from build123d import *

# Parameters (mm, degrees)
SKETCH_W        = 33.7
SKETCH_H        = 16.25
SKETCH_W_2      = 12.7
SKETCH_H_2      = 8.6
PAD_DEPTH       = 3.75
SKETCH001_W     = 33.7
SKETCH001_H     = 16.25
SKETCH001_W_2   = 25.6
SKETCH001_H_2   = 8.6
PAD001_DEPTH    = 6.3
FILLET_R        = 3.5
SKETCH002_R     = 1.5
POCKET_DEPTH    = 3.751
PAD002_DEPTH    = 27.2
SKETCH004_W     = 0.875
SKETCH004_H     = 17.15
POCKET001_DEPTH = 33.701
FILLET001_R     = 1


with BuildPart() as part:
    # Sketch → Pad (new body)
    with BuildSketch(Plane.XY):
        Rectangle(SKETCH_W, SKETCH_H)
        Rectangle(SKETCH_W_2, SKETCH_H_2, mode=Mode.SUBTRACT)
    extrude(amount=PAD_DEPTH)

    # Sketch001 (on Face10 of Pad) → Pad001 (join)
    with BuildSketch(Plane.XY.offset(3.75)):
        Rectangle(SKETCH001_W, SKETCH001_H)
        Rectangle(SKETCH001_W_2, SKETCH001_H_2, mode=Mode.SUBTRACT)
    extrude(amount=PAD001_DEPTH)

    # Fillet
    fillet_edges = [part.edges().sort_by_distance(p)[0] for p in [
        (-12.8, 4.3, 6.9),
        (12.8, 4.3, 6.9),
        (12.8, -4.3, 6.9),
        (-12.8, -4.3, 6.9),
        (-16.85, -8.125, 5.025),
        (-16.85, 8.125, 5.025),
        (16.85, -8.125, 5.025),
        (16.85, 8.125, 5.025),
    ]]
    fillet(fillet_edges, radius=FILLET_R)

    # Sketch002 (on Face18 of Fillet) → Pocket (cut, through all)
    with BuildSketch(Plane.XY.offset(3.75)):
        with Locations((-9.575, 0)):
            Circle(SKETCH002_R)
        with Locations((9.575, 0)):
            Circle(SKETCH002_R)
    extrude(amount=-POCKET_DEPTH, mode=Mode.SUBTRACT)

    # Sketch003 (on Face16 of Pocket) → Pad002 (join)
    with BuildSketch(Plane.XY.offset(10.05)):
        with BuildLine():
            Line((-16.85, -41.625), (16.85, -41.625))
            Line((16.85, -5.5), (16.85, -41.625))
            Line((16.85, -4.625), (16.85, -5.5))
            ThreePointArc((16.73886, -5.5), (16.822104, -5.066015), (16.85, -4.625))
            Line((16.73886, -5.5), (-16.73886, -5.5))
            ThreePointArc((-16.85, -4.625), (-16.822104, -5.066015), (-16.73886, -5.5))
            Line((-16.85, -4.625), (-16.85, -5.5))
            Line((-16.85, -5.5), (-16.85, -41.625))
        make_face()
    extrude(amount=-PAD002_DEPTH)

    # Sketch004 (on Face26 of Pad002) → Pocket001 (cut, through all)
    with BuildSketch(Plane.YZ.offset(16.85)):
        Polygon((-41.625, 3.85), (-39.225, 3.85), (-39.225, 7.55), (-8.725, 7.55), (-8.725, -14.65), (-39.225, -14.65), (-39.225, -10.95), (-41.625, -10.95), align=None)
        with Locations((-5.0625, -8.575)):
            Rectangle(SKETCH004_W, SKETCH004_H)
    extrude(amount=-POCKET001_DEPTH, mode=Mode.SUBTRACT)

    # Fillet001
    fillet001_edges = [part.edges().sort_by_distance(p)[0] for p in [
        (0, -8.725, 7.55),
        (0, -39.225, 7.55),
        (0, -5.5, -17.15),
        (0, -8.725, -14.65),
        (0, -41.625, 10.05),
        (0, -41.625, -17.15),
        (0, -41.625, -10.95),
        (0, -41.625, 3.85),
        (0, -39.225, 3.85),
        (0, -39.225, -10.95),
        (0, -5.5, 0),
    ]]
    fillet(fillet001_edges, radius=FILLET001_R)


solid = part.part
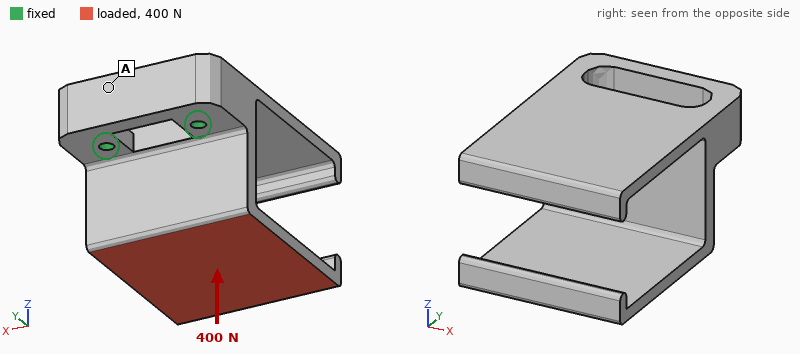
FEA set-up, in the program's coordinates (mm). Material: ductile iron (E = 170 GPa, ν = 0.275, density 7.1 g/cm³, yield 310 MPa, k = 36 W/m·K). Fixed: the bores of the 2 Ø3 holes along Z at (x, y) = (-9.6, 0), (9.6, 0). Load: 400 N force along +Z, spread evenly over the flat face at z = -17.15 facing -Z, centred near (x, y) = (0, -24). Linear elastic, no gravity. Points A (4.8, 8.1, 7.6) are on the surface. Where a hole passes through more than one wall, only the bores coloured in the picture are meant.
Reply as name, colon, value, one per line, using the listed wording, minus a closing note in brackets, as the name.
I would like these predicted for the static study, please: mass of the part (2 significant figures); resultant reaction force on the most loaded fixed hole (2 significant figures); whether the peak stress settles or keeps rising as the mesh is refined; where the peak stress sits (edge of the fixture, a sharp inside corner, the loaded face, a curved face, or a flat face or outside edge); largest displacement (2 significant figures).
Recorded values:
mass of the part: 84 g
resultant reaction force on the most loaded fixed hole: 210 N
whether the peak stress settles or keeps rising as the mesh is refined: keeps rising
where the peak stress sits: edge of the fixture
largest displacement: 0.50 mm
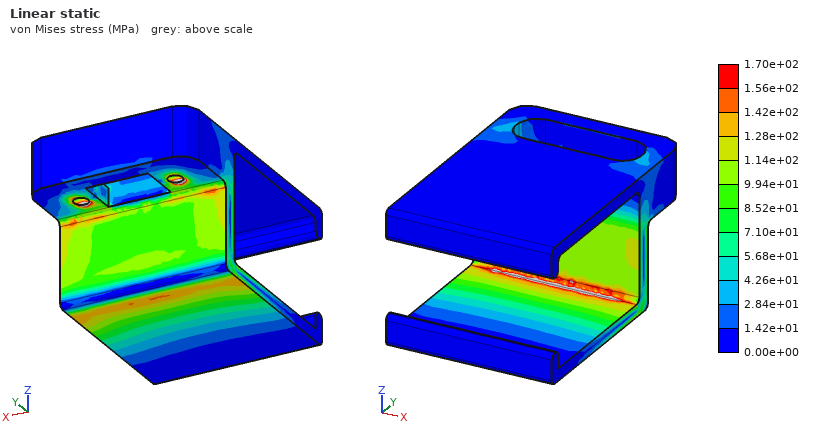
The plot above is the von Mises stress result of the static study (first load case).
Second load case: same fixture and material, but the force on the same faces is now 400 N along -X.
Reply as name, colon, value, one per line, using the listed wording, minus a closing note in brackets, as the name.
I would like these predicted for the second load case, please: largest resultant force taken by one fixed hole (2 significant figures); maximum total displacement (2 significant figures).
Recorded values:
largest resultant force taken by one fixed hole: 570 N
maximum total displacement: 88 µm
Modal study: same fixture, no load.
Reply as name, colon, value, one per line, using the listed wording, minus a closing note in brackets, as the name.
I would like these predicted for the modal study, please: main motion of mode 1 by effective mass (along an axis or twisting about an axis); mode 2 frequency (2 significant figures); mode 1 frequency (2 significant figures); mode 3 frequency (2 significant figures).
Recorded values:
main motion of mode 1 by effective mass: along Z
mode 2 frequency: 1400 Hz
mode 1 frequency: 1000 Hz
mode 3 frequency: 2300 Hz
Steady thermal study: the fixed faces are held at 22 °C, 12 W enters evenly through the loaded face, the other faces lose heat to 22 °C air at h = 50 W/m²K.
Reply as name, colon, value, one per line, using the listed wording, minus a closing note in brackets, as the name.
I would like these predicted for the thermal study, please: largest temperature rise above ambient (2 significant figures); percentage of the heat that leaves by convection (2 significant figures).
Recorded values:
largest temperature rise above ambient: 65 K
percentage of the heat that leaves by convection: 60 %
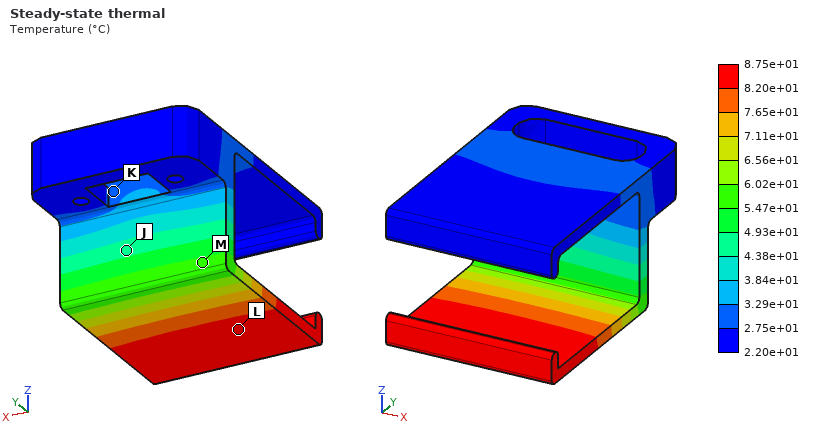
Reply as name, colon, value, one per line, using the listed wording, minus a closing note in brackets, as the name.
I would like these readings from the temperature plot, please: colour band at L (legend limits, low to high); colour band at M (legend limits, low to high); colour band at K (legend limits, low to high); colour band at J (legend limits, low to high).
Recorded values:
colour band at L: 8.20e+01 to 8.75e+01 °C
colour band at M: 5.47e+01 to 6.02e+01 °C
colour band at K: 2.75e+01 to 3.29e+01 °C
colour band at J: 4.38e+01 to 4.93e+01 °C
